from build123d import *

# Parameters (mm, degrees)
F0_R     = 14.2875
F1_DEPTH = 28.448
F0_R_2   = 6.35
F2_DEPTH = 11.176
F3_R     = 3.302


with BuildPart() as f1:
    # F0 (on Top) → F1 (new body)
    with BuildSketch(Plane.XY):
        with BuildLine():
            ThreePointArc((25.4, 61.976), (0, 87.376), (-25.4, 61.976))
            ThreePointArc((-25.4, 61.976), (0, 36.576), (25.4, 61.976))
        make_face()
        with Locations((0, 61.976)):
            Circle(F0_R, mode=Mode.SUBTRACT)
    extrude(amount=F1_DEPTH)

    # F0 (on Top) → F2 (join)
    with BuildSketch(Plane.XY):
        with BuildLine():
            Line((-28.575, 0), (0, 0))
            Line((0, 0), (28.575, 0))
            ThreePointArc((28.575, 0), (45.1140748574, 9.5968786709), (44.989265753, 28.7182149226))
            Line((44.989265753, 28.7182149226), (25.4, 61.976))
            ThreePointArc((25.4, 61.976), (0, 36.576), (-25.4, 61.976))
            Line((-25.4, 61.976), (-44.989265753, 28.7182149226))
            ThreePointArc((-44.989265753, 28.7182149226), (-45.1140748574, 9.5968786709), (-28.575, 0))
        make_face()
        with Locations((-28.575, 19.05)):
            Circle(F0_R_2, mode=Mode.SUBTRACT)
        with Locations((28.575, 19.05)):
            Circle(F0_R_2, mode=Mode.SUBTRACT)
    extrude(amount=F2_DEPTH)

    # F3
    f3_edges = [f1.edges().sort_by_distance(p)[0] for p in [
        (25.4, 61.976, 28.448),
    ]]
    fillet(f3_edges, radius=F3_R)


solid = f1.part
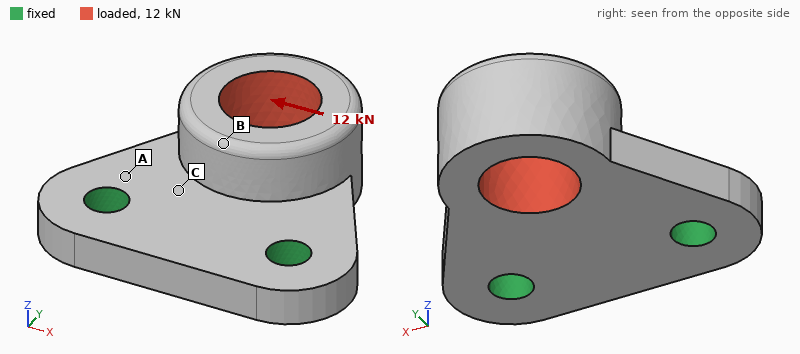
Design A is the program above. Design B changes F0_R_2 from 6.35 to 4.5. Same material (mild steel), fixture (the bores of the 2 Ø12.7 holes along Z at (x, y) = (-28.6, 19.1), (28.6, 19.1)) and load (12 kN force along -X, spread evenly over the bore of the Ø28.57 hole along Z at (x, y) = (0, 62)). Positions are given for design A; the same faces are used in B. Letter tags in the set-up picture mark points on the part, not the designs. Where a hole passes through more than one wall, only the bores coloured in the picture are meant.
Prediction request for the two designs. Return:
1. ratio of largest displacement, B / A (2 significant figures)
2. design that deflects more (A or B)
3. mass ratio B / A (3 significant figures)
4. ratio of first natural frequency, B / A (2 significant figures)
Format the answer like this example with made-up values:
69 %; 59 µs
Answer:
1.1; B; 1.02; 0.92
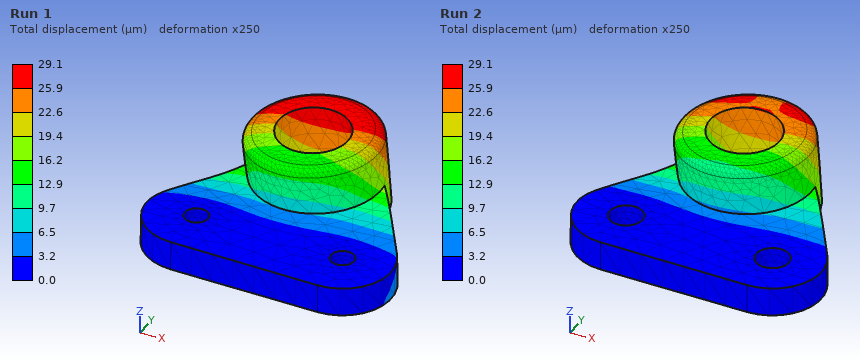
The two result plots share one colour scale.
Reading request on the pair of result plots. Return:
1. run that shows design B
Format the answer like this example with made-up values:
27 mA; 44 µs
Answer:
Run 1
